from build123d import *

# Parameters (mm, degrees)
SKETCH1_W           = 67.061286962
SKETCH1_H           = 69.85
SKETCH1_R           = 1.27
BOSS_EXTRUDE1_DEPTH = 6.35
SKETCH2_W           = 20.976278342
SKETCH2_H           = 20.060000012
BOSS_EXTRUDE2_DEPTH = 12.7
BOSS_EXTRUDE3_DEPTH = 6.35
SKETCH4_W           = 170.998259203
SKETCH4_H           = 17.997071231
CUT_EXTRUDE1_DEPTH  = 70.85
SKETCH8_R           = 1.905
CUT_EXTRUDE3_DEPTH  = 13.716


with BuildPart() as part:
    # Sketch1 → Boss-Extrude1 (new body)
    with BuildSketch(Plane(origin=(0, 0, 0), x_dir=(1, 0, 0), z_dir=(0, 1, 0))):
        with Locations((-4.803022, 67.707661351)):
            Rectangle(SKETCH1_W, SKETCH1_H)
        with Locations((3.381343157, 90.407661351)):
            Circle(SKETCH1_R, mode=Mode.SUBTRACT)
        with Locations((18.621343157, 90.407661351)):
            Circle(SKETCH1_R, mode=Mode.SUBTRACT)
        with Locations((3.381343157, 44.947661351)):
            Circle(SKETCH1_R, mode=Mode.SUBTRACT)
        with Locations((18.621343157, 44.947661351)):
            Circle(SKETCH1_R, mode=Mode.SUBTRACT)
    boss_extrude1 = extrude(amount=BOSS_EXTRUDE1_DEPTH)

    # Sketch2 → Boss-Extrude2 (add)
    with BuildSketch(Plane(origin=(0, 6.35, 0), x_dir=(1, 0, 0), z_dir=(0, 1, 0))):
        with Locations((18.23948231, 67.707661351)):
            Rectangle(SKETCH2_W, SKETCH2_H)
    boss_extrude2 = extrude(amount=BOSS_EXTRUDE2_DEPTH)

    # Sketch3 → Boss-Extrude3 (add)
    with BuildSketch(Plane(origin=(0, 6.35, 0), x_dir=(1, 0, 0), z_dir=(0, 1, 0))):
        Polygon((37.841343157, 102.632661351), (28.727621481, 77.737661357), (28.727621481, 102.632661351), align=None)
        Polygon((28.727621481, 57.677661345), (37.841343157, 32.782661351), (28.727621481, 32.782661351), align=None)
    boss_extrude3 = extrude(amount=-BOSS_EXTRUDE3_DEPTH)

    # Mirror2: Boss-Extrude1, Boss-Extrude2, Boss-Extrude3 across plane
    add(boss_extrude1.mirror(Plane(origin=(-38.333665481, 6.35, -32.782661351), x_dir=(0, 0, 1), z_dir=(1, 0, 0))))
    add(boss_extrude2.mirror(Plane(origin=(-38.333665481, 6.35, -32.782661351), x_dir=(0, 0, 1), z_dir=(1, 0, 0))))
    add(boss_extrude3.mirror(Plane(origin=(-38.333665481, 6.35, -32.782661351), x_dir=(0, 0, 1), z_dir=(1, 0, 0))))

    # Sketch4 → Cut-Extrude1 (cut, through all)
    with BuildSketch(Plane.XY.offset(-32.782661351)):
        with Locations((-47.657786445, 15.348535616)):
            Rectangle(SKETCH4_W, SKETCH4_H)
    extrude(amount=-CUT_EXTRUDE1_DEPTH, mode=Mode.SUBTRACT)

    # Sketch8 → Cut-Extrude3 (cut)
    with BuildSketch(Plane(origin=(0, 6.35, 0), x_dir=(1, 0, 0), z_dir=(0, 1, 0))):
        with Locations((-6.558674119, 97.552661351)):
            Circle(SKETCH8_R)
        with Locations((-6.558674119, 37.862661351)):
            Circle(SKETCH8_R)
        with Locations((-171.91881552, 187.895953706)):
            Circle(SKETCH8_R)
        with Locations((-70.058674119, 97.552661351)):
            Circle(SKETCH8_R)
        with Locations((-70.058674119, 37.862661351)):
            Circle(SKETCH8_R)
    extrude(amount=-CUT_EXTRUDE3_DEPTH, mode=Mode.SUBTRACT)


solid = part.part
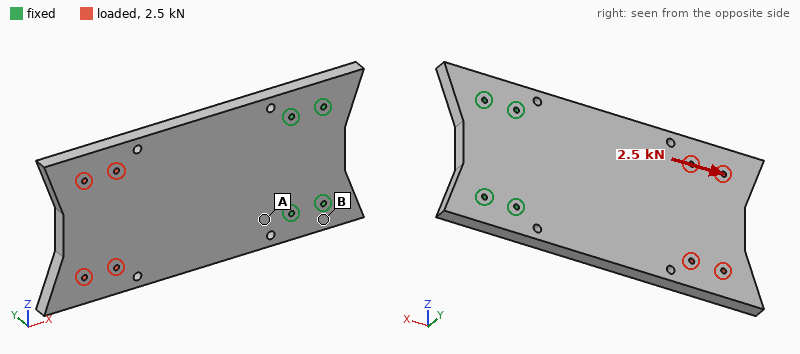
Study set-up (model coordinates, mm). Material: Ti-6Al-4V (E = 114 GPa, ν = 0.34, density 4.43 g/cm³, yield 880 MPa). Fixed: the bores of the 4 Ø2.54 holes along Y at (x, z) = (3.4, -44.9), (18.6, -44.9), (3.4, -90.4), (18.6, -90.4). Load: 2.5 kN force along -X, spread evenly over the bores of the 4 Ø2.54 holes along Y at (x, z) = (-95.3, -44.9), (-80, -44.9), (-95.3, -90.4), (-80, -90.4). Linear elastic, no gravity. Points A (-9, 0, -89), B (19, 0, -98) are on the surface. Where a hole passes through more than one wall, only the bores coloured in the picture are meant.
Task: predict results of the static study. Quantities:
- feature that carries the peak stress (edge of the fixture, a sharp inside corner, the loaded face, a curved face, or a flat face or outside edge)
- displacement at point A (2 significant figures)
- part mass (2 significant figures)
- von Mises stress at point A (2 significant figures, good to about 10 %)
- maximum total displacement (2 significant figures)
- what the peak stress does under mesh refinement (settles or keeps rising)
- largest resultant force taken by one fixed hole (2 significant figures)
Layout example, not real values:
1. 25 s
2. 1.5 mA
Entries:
1. edge of the fixture
2. 1.2 µm
3. 270 g
4. 7.7 MPa
5. 5.9 µm
6. keeps rising
7. 850 N
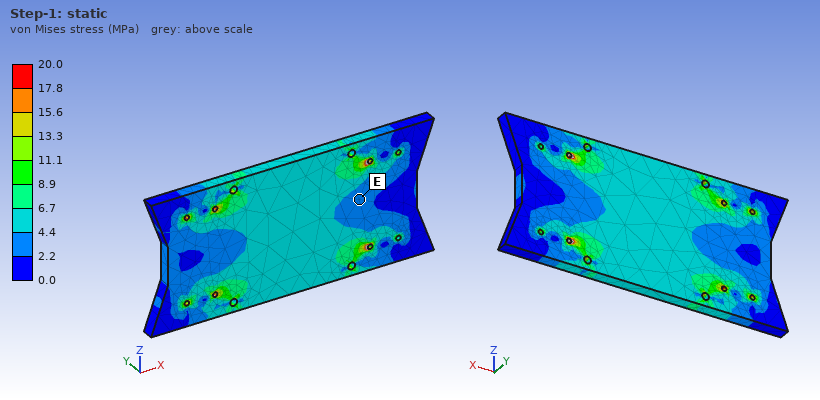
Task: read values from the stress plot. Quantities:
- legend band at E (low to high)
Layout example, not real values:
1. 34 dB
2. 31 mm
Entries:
1. 2.2 to 4.4 MPa
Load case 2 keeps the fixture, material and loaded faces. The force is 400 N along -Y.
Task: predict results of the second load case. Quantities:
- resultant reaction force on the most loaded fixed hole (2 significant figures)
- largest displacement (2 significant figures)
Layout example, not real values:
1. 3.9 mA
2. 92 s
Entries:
1. 850 N
2. 0.94 mm
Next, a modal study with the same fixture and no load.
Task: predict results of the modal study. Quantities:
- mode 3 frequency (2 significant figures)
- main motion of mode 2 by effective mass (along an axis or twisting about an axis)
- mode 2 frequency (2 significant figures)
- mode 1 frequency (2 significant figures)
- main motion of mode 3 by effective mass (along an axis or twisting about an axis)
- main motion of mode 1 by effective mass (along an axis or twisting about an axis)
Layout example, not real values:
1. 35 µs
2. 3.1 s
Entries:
1. 2400 Hz
2. twisting about X
3. 1400 Hz
4. 390 Hz
5. along Y
6. along Y
